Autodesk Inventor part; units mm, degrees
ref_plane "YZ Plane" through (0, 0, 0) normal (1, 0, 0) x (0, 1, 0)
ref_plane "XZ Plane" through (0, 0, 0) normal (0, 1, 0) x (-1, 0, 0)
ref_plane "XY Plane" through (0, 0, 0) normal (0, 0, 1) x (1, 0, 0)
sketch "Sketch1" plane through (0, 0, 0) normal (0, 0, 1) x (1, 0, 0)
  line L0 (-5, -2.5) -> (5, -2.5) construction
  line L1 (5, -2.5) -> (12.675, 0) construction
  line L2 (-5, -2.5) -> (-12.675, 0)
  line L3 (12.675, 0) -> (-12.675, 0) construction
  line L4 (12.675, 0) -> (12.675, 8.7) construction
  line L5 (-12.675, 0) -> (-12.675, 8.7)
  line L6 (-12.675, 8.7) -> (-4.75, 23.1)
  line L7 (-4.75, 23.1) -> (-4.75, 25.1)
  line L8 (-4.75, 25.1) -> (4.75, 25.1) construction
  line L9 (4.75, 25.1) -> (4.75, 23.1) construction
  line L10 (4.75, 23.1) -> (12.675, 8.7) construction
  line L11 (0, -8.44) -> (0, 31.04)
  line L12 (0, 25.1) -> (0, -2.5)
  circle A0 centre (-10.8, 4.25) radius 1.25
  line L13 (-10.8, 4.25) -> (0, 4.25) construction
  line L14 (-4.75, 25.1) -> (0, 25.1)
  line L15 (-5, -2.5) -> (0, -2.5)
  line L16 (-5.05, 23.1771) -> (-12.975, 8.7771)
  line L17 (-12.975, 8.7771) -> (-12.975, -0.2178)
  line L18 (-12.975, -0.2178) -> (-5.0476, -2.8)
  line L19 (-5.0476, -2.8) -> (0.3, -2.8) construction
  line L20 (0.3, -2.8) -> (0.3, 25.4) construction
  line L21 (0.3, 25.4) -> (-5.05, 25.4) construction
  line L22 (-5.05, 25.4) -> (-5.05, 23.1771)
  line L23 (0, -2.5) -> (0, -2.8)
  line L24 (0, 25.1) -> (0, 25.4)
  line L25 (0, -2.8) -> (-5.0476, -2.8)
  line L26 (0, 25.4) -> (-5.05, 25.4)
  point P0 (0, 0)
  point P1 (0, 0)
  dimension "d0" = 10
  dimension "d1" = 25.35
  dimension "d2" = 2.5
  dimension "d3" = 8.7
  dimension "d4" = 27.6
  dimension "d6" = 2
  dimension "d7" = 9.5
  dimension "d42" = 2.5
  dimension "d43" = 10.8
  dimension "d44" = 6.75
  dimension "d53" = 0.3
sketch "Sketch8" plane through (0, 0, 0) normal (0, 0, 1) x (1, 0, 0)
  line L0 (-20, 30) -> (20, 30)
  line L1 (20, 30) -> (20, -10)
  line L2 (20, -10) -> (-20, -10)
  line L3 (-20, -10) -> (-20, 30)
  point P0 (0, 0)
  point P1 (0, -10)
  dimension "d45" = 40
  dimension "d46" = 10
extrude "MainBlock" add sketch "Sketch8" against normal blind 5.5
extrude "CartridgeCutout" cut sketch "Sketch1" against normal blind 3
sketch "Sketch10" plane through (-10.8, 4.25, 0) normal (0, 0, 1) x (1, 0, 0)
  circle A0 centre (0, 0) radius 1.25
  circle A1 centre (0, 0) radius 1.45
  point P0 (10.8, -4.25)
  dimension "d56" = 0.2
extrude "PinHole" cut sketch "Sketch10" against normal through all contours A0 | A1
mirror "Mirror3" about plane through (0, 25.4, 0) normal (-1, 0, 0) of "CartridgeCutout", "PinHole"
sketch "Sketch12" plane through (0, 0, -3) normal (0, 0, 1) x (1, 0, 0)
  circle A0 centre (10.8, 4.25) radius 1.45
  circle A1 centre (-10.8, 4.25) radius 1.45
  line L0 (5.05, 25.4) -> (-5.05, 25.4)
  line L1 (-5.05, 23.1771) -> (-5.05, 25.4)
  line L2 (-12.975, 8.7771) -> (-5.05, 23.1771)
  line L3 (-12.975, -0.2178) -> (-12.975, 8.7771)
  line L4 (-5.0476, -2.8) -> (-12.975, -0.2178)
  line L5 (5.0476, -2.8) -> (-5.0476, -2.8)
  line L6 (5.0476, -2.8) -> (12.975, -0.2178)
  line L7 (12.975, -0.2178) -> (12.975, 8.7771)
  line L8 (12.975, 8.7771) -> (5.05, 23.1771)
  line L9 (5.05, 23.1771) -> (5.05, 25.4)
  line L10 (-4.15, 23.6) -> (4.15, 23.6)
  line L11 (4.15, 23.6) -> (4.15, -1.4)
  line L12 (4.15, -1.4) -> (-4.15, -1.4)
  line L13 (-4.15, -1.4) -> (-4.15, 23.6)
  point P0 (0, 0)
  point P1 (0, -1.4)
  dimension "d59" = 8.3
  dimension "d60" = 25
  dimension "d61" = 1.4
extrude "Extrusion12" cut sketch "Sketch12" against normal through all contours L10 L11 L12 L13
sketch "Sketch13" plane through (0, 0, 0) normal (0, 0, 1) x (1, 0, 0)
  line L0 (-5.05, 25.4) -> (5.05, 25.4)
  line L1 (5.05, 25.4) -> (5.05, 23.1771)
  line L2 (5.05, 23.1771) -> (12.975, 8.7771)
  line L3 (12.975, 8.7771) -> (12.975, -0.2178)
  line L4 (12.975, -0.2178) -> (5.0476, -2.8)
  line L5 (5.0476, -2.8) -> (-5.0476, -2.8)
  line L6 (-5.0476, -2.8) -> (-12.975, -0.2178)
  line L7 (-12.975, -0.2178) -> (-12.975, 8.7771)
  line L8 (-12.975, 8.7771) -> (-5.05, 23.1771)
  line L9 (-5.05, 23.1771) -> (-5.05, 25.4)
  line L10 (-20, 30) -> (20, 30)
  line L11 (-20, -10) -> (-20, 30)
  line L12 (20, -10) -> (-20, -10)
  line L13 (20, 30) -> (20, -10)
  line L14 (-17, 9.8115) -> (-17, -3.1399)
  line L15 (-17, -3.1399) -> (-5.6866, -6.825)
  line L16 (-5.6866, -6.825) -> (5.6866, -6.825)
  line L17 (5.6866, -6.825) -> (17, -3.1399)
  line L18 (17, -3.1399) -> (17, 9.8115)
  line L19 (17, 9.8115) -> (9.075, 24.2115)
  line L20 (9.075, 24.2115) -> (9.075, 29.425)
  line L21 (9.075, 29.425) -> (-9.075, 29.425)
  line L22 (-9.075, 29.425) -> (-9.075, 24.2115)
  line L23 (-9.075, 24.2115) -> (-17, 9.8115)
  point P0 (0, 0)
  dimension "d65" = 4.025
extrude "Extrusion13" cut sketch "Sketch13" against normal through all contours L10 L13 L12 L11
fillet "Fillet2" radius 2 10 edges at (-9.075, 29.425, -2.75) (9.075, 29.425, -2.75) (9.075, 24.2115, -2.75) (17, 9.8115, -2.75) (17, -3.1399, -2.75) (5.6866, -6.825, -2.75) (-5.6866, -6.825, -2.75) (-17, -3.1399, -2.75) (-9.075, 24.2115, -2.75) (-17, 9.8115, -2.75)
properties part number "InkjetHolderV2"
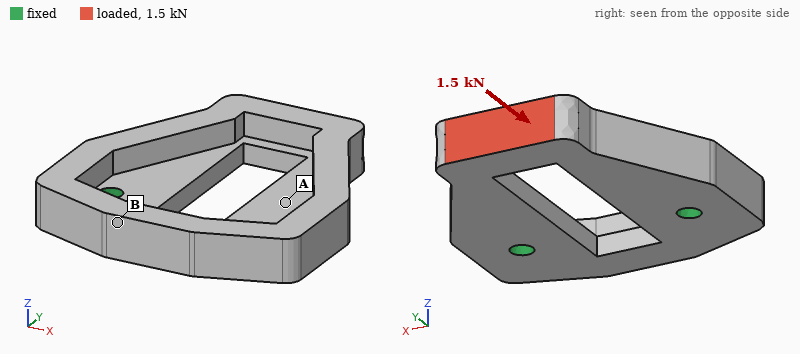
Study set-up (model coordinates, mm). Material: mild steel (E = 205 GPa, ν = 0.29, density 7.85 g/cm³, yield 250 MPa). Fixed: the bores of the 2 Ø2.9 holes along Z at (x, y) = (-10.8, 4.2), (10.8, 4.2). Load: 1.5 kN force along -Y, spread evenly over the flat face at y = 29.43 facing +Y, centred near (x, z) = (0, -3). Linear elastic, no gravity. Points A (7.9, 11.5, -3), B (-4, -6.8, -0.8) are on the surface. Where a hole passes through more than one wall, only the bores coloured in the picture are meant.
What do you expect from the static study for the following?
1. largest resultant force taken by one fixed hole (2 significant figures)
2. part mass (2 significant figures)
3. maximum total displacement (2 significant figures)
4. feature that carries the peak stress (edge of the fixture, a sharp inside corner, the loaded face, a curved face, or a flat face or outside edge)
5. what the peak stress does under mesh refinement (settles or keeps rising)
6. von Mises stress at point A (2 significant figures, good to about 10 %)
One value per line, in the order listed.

820 N
25 g
27 µm
edge of the fixture
keeps rising
39 MPa
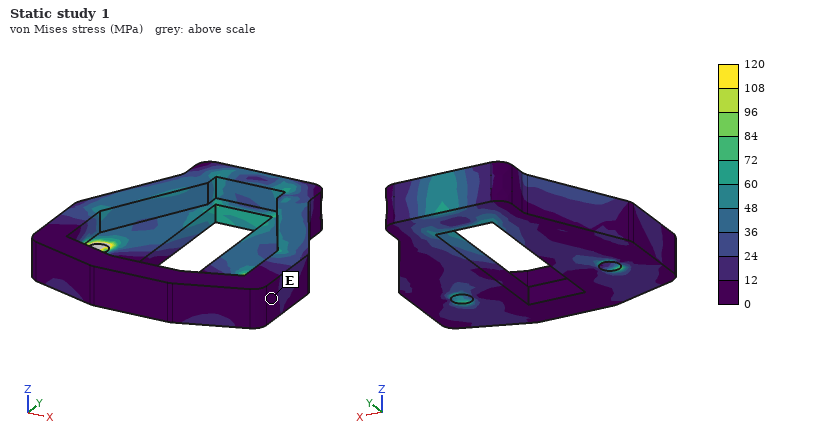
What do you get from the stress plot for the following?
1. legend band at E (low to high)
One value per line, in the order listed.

0 to 12 MPa
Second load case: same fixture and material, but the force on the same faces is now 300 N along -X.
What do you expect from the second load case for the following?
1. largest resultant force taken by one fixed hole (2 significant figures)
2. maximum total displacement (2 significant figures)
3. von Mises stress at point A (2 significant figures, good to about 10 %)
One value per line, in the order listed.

290 N
7.0 µm
11 MPa
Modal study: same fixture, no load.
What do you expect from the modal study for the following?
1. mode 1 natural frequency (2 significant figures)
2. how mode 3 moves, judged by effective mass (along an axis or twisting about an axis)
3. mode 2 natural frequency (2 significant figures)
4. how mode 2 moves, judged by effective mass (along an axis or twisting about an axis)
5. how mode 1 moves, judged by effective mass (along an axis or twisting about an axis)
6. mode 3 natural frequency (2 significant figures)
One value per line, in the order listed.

4500 Hz
along X
11 kHz
along X
along Z
13 kHz
